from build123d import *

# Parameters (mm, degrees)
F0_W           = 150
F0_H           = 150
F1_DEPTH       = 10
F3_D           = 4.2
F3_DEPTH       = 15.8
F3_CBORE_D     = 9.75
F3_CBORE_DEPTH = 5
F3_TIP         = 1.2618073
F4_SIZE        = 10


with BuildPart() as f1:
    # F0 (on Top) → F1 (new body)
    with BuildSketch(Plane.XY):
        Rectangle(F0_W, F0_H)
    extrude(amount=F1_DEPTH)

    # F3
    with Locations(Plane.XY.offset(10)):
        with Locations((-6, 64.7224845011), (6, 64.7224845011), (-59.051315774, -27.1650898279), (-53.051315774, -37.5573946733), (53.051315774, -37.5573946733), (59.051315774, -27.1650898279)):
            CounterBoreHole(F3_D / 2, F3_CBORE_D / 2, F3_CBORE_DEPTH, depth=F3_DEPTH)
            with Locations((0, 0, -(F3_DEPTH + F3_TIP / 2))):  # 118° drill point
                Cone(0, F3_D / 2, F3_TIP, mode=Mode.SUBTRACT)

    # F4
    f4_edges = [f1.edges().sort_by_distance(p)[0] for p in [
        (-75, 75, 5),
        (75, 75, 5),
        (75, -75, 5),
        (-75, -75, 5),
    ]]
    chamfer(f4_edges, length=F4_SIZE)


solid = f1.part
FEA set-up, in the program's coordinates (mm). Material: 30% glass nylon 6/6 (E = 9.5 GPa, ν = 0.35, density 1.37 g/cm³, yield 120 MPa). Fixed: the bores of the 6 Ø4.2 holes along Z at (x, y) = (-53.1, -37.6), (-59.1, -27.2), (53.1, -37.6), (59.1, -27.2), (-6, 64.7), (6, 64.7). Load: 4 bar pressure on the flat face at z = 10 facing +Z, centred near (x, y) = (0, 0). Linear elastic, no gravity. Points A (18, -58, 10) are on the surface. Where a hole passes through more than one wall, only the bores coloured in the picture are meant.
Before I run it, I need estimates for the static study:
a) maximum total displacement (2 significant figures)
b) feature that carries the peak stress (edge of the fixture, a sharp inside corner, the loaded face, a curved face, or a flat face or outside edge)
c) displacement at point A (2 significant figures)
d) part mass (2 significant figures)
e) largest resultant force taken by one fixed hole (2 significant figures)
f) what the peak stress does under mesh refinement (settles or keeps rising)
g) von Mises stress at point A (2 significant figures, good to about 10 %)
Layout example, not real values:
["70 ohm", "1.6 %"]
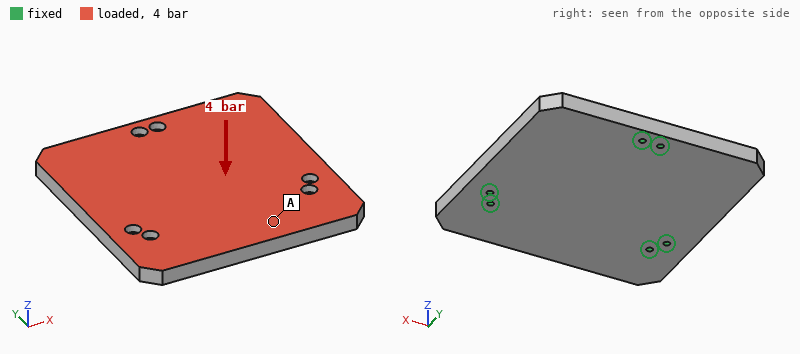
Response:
["1.0 mm", "edge of the fixture", "0.40 mm", "300 g", "2.1 kN", "keeps rising", "14 MPa"]
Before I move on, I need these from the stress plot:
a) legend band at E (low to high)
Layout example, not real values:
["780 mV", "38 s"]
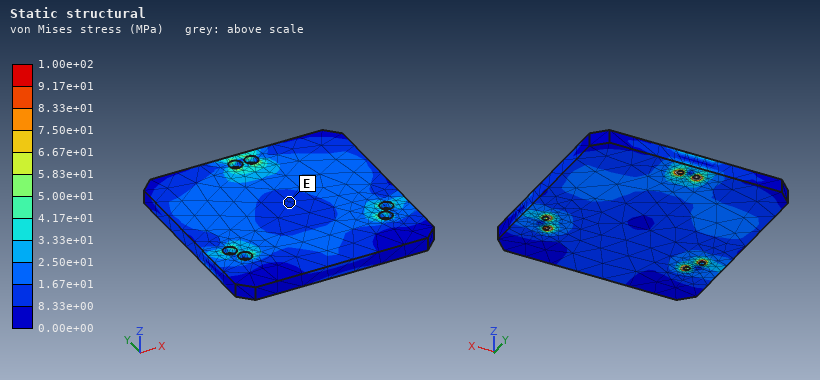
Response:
["8.33e+00 to 1.67e+01 MPa"]
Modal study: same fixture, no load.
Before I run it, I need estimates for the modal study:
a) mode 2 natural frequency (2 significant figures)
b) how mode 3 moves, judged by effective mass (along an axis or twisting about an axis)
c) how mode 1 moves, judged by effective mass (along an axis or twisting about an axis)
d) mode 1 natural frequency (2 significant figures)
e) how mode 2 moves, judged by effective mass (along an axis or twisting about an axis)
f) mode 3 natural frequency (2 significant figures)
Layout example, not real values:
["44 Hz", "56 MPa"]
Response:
["1100 Hz", "along Z", "twisting about Y", "960 Hz", "along Z", "1400 Hz"]
